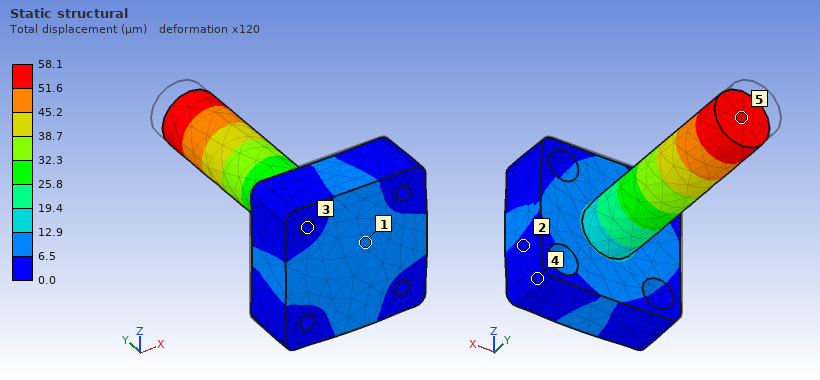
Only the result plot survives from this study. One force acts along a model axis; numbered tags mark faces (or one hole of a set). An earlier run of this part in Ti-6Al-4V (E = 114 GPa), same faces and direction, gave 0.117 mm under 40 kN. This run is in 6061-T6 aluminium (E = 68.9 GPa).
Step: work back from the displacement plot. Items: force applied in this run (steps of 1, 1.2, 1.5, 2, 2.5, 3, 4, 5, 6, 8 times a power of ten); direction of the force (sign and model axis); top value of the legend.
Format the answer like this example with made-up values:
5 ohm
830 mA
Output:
12 kN
-Y
58.1 µm
